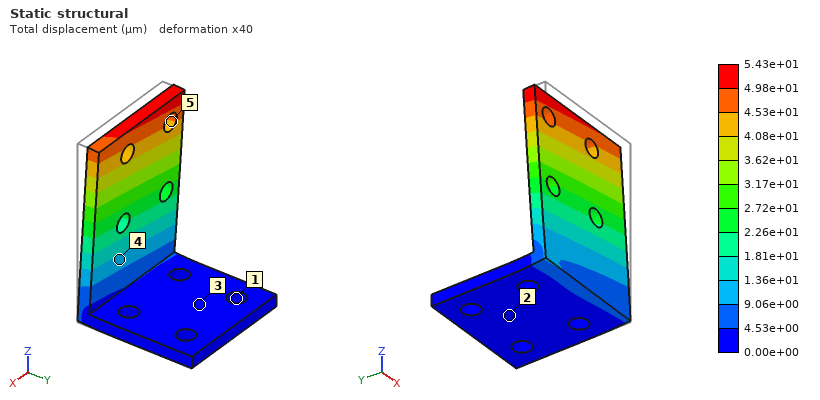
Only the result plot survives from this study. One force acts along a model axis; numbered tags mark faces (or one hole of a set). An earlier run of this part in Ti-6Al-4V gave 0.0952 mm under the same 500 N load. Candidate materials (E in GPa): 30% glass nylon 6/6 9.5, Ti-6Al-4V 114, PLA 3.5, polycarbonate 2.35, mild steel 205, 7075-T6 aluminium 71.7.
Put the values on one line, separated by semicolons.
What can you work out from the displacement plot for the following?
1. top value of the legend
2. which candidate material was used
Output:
5.43e+01 µm; mild steel
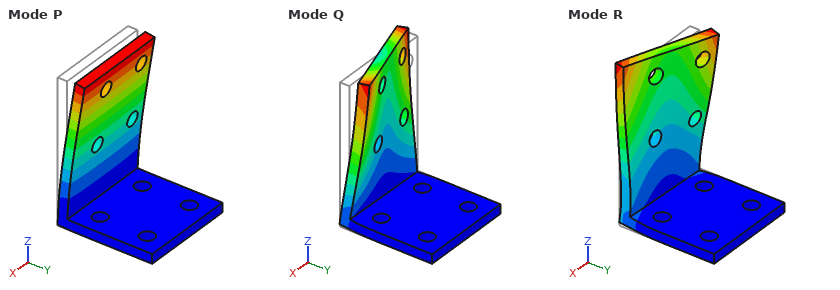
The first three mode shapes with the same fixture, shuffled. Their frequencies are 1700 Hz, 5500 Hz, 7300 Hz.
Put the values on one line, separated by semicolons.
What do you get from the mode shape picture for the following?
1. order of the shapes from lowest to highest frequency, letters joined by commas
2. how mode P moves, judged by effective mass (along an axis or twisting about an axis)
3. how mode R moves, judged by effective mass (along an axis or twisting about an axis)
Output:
P, Q, R; along Y; along X
